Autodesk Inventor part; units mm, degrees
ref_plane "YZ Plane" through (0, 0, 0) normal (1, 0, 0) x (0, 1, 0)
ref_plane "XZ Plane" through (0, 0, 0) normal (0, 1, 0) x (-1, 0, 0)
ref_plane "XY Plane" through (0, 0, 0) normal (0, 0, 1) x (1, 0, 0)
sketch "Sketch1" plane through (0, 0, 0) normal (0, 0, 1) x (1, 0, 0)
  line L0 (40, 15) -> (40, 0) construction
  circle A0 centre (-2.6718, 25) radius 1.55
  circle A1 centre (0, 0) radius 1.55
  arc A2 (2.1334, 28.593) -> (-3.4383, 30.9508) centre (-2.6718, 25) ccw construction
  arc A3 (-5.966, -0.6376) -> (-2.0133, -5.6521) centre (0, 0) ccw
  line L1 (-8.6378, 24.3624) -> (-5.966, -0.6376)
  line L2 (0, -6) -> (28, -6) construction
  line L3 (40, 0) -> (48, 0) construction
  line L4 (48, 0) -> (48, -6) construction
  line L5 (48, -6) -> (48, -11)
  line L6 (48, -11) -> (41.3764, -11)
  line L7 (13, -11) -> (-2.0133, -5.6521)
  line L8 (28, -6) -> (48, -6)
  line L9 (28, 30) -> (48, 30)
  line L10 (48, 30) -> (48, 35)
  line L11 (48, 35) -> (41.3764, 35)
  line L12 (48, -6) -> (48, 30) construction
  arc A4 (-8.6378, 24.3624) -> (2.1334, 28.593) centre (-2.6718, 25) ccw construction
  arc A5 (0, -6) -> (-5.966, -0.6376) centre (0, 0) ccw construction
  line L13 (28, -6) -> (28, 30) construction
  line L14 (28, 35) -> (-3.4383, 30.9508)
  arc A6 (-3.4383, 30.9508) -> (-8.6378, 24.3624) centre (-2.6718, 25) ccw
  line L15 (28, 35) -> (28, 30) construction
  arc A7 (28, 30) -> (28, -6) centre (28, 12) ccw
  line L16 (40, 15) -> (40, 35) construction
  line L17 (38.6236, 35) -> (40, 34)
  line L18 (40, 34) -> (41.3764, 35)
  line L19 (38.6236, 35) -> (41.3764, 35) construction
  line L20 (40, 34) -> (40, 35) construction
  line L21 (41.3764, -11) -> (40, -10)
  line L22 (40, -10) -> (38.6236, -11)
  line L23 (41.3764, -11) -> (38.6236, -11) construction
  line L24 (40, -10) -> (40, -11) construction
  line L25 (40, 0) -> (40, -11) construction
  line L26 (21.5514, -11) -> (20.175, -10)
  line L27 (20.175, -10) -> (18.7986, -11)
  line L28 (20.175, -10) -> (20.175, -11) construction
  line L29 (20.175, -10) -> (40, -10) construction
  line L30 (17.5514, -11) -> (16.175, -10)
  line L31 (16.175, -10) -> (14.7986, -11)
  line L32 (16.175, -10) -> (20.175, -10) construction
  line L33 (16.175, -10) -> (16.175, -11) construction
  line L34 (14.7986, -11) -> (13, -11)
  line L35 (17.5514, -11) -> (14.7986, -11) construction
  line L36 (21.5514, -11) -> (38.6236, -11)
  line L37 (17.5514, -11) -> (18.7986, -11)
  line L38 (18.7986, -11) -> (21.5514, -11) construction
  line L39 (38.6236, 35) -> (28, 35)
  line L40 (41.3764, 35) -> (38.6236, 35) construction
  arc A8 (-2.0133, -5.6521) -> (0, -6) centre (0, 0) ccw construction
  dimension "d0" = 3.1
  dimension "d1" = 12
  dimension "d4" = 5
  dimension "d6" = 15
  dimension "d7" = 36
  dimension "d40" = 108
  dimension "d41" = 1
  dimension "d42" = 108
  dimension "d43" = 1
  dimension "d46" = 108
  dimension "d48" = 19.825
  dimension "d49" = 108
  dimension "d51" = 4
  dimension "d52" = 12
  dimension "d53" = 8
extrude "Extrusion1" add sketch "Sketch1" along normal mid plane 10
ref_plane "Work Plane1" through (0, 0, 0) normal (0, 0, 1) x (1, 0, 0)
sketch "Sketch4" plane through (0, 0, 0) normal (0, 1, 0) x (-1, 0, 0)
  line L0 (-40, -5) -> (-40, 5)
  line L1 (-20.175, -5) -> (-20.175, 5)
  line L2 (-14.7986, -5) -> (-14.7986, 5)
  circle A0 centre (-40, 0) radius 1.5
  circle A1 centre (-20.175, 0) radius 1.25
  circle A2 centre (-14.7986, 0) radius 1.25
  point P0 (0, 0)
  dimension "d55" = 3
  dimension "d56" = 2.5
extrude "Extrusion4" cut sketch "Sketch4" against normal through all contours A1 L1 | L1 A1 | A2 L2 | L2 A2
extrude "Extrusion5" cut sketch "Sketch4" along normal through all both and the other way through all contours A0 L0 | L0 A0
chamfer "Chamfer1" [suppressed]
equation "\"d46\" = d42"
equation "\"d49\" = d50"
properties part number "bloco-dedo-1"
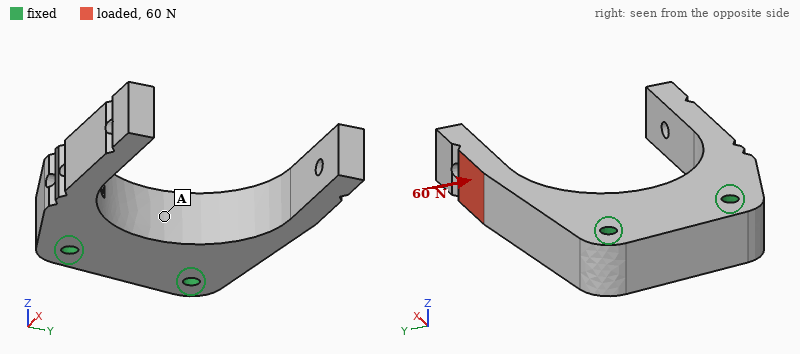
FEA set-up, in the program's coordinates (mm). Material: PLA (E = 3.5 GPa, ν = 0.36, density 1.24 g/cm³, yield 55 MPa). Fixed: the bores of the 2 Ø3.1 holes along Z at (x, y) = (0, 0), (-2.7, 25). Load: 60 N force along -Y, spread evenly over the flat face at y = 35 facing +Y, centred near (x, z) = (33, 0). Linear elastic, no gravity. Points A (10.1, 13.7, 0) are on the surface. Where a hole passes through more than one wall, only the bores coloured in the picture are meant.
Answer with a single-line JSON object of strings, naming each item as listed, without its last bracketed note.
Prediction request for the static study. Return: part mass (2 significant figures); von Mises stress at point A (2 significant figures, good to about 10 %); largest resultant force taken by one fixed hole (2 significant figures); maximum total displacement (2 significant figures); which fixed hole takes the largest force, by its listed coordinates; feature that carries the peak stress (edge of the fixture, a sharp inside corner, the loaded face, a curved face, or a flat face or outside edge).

{"part mass": "14 g", "von Mises stress at point A": "2.7 MPa", "largest resultant force taken by one fixed hole": "110 N", "maximum total displacement": "0.76 mm", "which fixed hole takes the largest force, by its listed coordinates": "(0, 0)", "feature that carries the peak stress": "a curved face"}
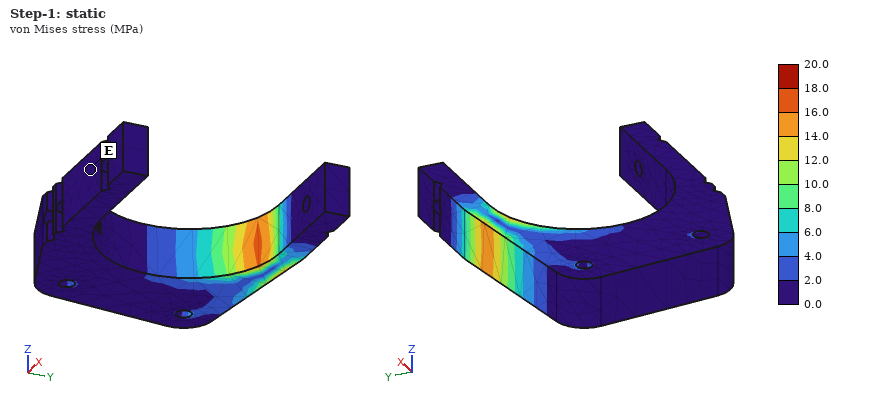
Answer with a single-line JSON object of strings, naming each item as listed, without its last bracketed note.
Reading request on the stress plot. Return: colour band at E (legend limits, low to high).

{"colour band at E": "0.0 to 2.0 MPa"}
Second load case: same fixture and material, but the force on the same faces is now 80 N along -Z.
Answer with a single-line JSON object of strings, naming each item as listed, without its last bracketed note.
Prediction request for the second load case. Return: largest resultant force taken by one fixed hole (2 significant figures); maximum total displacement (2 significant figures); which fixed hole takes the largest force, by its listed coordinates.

{"largest resultant force taken by one fixed hole": "93 N", "maximum total displacement": "0.77 mm", "which fixed hole takes the largest force, by its listed coordinates": "(-2.7, 25)"}
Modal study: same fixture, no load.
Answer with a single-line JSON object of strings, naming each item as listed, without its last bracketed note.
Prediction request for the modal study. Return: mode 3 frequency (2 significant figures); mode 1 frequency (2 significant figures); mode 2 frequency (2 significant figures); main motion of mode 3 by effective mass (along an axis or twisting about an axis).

{"mode 3 frequency": "1400 Hz", "mode 1 frequency": "1300 Hz", "mode 2 frequency": "1300 Hz", "main motion of mode 3 by effective mass": "along Z"}
